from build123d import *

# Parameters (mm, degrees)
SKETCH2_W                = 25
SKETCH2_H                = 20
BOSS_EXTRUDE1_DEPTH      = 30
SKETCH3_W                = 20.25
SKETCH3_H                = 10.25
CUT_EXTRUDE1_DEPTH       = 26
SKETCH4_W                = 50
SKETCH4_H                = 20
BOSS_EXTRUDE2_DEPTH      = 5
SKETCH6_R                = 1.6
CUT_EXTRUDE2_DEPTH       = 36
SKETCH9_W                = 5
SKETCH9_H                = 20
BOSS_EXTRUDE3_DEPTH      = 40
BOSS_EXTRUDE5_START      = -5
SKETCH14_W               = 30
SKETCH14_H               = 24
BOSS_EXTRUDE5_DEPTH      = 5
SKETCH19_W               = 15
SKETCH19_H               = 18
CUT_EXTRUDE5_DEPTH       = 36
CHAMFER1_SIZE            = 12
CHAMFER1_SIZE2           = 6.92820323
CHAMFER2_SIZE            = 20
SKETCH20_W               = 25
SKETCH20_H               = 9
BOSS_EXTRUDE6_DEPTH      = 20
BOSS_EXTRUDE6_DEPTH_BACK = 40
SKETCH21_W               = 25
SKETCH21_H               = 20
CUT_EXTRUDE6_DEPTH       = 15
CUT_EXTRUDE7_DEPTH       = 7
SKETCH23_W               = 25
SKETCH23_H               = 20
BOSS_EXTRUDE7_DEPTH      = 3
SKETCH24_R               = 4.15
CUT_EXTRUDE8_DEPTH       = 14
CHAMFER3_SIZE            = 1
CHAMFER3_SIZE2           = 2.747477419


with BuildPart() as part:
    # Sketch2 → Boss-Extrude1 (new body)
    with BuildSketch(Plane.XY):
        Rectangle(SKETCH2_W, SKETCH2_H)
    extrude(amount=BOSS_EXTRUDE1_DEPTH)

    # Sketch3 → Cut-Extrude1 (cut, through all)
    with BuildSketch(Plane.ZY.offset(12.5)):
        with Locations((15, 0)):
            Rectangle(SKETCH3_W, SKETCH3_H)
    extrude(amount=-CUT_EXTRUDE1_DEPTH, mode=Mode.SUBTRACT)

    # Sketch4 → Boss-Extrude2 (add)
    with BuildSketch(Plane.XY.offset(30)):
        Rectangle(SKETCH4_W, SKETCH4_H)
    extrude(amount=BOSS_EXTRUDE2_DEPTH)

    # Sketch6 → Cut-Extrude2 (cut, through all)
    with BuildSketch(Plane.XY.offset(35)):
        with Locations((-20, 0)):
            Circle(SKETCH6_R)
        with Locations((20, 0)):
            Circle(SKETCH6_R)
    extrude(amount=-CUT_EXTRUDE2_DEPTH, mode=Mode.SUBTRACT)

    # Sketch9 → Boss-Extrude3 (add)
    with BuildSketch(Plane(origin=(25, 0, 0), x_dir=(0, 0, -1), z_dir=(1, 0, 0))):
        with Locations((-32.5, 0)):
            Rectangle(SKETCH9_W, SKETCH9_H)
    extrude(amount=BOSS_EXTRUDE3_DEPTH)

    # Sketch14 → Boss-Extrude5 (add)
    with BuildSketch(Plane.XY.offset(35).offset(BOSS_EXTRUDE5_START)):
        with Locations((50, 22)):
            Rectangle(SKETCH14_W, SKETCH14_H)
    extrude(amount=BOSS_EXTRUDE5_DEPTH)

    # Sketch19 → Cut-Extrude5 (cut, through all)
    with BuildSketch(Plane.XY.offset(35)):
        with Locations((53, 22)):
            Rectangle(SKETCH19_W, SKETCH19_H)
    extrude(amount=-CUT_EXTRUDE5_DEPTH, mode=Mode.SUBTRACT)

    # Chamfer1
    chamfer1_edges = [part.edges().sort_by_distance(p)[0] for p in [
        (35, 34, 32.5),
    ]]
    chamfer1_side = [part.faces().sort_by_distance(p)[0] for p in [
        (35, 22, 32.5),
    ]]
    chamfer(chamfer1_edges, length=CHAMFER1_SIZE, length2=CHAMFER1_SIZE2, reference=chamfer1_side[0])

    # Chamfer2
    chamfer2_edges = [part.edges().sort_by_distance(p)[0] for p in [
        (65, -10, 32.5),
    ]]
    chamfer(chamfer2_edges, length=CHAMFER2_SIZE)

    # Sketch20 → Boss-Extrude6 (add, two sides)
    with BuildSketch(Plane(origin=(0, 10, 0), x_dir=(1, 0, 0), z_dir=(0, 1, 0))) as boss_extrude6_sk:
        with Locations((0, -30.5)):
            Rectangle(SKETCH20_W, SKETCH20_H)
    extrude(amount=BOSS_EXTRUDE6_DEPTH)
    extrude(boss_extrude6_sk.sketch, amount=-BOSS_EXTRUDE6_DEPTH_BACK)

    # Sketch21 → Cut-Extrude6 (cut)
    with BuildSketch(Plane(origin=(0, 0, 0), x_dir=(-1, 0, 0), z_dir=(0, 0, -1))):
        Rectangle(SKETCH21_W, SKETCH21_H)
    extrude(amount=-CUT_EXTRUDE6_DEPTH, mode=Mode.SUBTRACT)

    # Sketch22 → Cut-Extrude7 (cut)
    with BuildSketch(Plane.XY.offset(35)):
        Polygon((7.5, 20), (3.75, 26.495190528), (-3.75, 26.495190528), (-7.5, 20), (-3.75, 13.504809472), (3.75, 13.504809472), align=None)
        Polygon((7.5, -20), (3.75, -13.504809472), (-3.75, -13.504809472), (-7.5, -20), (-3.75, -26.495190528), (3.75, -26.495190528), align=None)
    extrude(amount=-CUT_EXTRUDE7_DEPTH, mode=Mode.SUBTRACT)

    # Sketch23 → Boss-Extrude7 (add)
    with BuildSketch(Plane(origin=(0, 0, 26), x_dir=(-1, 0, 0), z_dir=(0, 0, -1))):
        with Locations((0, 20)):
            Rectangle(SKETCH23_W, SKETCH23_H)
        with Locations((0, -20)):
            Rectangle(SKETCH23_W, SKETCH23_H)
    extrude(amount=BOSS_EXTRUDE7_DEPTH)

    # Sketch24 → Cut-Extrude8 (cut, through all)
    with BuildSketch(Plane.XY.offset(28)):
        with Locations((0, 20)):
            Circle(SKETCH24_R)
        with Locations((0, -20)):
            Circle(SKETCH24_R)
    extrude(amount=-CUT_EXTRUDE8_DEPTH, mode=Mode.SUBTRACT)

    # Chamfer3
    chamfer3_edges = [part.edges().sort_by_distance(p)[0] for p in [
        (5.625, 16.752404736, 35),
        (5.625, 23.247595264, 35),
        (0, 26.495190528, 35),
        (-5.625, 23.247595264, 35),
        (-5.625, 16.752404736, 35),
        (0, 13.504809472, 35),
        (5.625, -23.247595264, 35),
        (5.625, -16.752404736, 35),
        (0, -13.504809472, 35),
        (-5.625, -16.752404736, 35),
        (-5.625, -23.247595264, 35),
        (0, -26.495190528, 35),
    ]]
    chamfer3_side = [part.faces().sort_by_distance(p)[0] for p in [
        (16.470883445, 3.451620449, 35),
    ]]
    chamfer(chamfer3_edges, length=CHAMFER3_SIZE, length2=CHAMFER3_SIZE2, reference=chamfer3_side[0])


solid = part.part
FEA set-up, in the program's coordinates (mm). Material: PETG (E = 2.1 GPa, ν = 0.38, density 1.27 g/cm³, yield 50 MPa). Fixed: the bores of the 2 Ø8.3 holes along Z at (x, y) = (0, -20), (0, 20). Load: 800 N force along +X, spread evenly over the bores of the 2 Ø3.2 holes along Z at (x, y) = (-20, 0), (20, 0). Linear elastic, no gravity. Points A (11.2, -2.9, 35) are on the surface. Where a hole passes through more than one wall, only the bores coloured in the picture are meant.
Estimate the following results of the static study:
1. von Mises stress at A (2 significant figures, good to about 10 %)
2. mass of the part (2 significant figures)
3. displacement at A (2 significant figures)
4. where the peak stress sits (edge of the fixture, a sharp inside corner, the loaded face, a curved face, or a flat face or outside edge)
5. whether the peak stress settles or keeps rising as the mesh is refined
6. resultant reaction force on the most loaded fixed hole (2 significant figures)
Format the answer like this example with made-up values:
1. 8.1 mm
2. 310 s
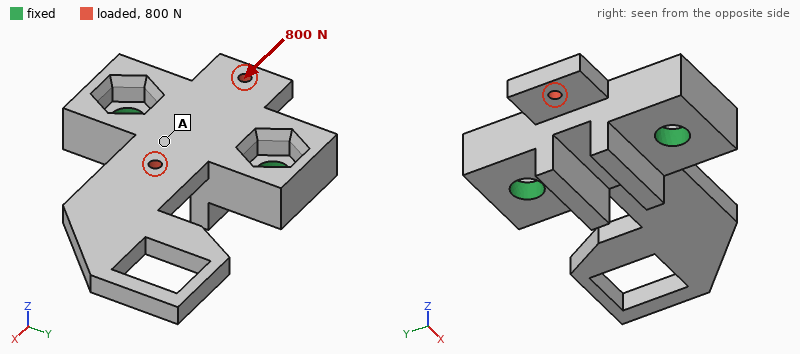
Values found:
1. 3.9 MPa
2. 31 g
3. 0.19 mm
4. edge of the fixture
5. keeps rising
6. 400 N
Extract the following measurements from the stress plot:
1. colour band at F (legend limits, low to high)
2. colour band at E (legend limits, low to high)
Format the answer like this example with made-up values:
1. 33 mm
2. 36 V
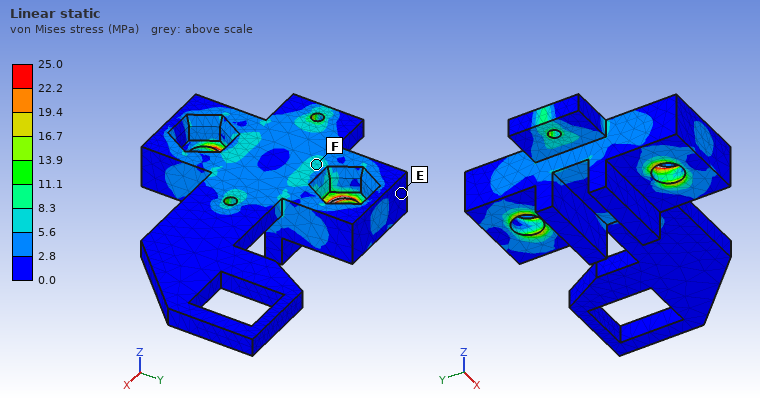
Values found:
1. 5.6 to 8.3 MPa
2. 0.0 to 2.8 MPa
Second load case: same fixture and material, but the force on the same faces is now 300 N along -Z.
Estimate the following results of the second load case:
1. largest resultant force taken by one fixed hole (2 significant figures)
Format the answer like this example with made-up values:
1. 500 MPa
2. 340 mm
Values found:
1. 230 N
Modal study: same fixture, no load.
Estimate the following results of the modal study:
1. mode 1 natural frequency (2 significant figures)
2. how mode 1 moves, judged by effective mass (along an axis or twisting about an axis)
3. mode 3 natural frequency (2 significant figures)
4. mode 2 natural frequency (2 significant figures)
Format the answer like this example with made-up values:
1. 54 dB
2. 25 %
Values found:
1. 280 Hz
2. along Z
3. 920 Hz
4. 790 Hz
